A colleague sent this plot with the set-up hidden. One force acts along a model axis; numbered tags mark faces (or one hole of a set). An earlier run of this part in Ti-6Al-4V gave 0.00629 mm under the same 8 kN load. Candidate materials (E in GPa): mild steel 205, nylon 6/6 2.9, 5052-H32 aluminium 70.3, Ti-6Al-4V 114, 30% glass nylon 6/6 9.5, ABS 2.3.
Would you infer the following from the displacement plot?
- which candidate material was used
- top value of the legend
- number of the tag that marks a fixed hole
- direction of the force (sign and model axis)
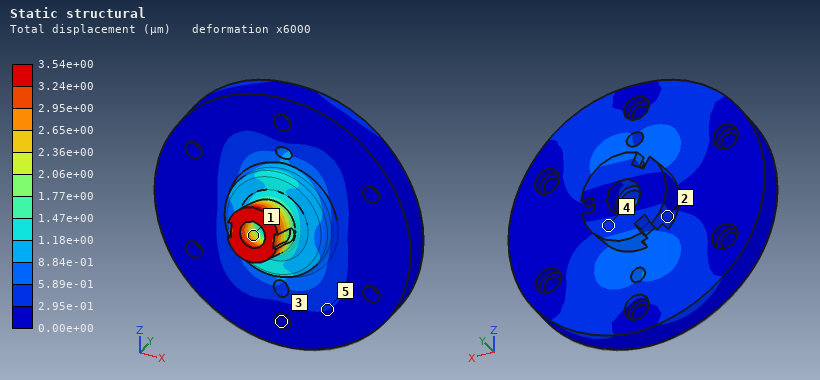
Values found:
mild steel
3.54e+00 µm
3
+Z
